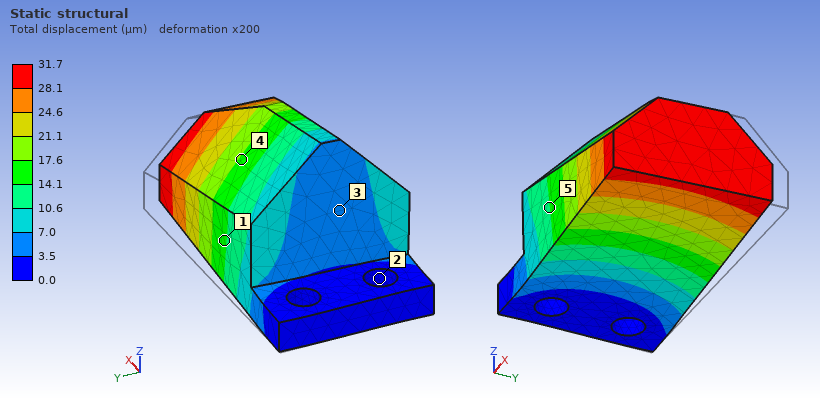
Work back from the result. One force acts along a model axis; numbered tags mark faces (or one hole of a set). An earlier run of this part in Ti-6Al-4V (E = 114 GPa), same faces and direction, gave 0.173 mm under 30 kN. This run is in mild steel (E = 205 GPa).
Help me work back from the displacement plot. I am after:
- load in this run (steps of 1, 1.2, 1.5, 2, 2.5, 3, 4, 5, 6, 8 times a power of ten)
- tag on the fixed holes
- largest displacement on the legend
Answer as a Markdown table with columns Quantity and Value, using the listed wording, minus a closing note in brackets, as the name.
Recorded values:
| Quantity | Value |
|---|---|
| load in this run | 10 kN |
| tag on the fixed holes | 2 |
| largest displacement on the legend | 31.7 µm |
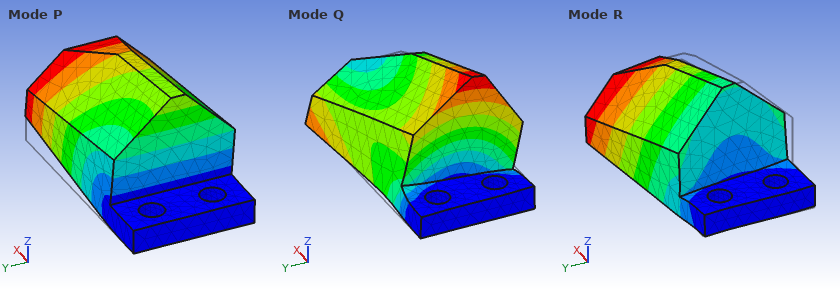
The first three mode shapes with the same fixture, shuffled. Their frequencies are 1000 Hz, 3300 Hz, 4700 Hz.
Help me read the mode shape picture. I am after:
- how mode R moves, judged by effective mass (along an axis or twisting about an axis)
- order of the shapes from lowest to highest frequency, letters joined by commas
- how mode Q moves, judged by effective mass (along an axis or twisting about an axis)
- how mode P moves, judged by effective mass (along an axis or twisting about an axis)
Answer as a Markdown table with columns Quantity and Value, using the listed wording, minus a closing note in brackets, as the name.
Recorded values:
| Quantity | Value |
|---|---|
| how mode R moves, judged by effective mass | along Y |
| order of the shapes from lowest to highest frequency, letters joined by commas | P, R, Q |
| how mode Q moves, judged by effective mass | twisting about X |
| how mode P moves, judged by effective mass | along Z |
